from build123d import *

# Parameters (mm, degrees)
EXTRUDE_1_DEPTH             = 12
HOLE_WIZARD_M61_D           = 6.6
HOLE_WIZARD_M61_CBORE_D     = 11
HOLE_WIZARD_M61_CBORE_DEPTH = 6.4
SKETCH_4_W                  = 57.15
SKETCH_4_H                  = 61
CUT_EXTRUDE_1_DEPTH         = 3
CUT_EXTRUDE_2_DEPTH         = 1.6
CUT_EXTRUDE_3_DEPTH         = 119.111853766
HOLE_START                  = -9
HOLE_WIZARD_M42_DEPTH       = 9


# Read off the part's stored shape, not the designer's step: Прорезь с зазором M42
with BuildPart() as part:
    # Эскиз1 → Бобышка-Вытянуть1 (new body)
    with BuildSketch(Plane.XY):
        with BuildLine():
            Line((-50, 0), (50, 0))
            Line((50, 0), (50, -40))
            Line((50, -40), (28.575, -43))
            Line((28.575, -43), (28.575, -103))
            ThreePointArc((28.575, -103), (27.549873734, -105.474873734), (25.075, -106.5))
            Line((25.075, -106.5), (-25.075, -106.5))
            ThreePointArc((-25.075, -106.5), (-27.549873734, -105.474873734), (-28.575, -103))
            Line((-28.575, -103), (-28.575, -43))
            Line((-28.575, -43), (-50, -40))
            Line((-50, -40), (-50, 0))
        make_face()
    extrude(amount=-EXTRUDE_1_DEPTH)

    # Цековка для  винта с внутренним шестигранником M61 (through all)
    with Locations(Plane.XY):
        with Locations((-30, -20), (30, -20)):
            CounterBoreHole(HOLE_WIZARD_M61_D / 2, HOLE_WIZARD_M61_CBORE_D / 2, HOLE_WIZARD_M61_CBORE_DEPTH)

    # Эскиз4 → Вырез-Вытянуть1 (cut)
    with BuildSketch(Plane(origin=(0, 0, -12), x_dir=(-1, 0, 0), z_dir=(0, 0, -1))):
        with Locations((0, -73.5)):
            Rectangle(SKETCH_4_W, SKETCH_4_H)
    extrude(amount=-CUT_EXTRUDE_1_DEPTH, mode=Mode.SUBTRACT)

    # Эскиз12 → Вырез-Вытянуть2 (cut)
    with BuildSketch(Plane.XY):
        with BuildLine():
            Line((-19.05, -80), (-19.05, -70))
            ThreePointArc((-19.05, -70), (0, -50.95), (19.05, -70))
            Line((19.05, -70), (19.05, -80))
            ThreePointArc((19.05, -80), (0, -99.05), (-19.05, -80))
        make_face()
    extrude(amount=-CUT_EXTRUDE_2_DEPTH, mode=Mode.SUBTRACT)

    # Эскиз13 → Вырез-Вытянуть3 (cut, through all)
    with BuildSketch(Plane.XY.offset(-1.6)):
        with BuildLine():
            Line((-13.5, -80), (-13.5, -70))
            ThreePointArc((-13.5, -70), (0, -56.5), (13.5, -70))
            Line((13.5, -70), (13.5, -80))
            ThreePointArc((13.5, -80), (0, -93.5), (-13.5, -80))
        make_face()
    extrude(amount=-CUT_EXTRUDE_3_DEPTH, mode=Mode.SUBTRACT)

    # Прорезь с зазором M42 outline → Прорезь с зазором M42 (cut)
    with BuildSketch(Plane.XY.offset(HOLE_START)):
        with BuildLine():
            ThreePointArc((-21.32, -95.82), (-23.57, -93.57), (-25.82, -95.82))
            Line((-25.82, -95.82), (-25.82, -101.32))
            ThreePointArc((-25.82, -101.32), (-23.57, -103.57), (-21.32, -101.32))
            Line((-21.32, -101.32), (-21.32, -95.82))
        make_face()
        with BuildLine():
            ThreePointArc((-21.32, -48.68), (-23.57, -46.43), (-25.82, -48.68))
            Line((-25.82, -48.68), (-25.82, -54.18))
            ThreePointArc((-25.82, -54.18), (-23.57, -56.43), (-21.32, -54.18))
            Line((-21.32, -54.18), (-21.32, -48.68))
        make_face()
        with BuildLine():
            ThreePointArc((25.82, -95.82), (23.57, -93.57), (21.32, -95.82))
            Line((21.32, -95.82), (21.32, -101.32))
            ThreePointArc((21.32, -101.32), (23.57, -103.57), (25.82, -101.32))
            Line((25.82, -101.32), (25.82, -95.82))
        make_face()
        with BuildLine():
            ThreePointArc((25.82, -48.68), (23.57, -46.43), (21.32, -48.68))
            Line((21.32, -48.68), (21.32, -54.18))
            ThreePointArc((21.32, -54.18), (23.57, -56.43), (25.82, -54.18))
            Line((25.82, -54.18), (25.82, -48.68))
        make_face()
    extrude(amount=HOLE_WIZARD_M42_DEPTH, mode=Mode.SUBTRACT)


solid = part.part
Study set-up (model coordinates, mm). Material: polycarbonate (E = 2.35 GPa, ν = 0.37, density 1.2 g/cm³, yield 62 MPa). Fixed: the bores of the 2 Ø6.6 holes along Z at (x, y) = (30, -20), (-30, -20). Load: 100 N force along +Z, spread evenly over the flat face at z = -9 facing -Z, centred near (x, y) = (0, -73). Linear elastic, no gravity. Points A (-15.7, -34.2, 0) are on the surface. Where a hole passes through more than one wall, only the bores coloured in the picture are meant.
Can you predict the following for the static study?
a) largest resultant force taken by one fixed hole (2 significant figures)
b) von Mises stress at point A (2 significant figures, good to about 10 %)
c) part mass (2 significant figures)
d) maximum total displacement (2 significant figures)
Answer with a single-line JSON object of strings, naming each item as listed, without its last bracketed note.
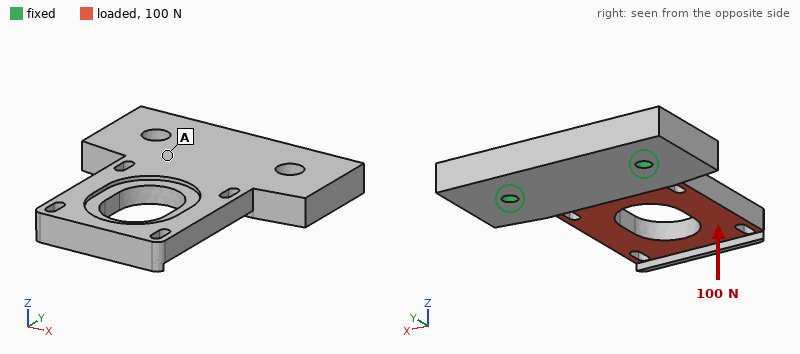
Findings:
{"largest resultant force taken by one fixed hole": "77 N", "von Mises stress at point A": "2.6 MPa", "part mass": "87 g", "maximum total displacement": "1.5 mm"}
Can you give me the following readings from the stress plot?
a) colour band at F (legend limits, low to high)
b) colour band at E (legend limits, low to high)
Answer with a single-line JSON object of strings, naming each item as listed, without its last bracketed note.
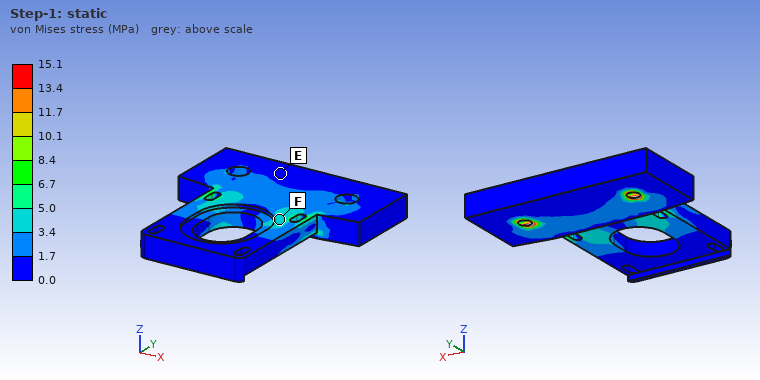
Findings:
{"colour band at F": "3.4 to 5.0 MPa", "colour band at E": "0.0 to 1.7 MPa"}
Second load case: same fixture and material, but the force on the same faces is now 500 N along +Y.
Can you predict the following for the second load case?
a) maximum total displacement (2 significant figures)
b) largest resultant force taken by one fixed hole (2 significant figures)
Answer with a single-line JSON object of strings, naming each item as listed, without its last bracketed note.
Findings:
{"maximum total displacement": "0.72 mm", "largest resultant force taken by one fixed hole": "260 N"}
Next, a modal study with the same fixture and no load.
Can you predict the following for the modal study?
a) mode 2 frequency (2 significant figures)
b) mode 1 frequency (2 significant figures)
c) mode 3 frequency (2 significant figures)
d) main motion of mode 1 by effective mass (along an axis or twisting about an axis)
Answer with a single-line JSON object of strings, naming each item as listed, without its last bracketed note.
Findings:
{"mode 2 frequency": "810 Hz", "mode 1 frequency": "280 Hz", "mode 3 frequency": "1200 Hz", "main motion of mode 1 by effective mass": "along Z"}
